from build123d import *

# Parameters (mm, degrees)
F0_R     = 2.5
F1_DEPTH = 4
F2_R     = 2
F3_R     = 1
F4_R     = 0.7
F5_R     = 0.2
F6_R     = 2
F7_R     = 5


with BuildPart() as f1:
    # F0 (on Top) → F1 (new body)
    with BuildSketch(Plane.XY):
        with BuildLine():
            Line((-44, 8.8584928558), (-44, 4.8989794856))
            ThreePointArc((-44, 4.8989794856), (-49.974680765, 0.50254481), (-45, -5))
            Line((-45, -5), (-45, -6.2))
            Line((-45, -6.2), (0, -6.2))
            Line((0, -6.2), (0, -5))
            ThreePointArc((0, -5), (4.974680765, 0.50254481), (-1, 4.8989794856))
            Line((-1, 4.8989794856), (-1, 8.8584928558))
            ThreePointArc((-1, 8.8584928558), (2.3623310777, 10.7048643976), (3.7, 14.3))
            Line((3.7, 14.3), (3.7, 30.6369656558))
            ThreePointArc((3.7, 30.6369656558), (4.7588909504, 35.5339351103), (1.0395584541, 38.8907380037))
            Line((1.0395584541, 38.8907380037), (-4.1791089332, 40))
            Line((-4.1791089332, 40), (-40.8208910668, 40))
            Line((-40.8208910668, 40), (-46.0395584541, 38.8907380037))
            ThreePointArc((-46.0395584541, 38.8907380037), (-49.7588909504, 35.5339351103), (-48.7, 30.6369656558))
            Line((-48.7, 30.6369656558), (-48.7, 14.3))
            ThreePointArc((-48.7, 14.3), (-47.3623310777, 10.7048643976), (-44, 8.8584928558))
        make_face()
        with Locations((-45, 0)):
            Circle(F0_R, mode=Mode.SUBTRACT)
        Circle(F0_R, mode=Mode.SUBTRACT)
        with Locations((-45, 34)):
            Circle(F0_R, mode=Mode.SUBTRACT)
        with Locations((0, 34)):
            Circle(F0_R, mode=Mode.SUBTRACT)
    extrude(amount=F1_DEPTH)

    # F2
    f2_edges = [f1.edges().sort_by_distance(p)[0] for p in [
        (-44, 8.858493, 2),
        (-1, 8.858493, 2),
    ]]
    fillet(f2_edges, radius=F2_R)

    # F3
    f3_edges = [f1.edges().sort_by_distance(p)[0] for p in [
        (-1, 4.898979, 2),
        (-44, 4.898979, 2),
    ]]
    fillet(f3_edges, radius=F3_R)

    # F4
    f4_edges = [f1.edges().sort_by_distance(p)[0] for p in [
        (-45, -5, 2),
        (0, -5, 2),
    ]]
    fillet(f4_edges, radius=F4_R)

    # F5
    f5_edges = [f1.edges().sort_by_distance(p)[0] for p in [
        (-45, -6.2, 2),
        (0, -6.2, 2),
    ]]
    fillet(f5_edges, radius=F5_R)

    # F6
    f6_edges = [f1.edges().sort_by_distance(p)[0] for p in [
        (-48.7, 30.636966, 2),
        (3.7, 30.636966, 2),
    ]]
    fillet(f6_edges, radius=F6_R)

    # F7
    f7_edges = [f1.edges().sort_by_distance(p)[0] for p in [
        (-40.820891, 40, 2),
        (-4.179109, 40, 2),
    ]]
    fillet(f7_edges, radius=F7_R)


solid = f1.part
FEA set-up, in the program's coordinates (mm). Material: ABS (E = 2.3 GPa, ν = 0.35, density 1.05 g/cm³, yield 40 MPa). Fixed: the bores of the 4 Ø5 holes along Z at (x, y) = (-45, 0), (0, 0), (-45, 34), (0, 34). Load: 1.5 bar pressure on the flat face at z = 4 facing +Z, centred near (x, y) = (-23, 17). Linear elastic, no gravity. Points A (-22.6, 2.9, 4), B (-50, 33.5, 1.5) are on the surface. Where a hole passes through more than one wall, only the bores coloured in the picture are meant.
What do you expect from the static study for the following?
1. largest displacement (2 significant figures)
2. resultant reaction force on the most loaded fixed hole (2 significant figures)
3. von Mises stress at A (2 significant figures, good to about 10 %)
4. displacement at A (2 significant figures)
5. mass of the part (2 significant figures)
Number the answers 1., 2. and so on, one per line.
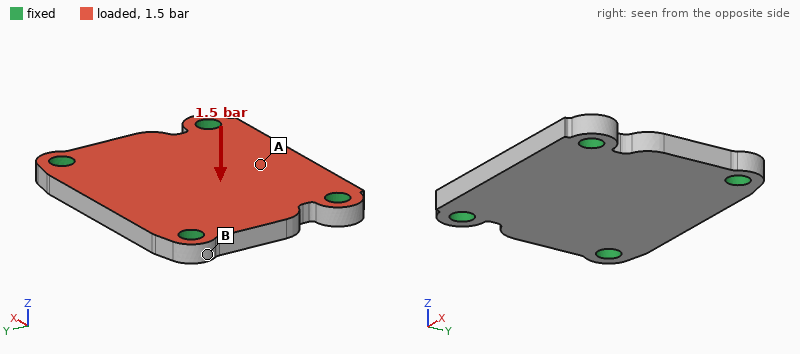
1. 0.18 mm
2. 88 N
3. 4.6 MPa
4. 0.15 mm
5. 9.6 g
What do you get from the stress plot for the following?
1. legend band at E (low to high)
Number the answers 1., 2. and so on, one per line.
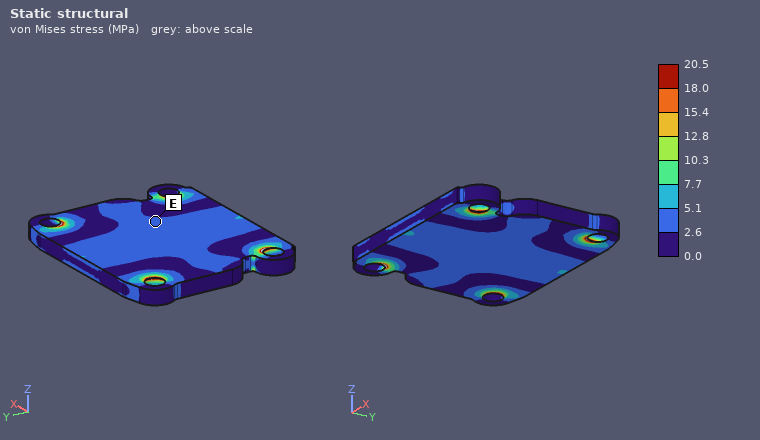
1. 2.6 to 5.1 MPa
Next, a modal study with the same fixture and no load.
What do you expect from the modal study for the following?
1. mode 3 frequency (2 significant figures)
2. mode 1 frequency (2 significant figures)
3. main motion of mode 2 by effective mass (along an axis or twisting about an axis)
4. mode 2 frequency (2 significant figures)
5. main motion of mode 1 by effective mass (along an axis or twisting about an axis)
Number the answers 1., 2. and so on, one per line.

1. 4600 Hz
2. 2600 Hz
3. twisting about X
4. 3700 Hz
5. along Z
